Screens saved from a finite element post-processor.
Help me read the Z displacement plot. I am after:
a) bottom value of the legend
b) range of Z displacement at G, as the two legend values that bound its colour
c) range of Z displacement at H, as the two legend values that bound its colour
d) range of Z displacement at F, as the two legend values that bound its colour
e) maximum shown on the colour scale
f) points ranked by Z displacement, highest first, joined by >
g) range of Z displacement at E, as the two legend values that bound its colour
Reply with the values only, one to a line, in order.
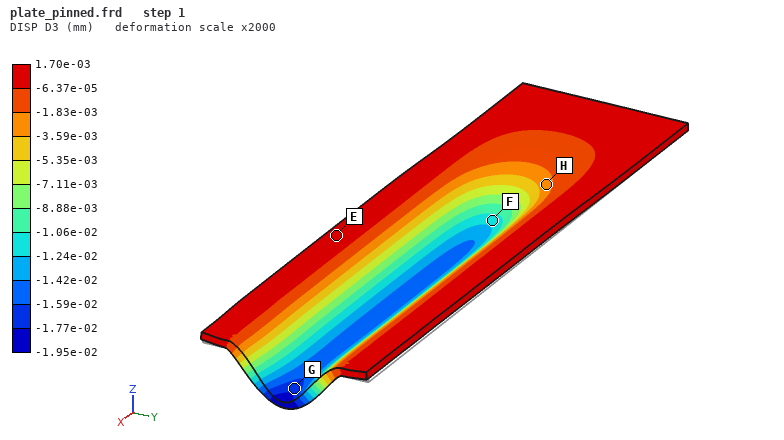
-1.95e-02 mm
-1.77e-02 to -1.59e-02 mm
-3.59e-03 to -1.83e-03 mm
-1.24e-02 to -1.06e-02 mm
1.70e-03 mm
E > H > F > G
-6.37e-05 to 1.70e-03 mm
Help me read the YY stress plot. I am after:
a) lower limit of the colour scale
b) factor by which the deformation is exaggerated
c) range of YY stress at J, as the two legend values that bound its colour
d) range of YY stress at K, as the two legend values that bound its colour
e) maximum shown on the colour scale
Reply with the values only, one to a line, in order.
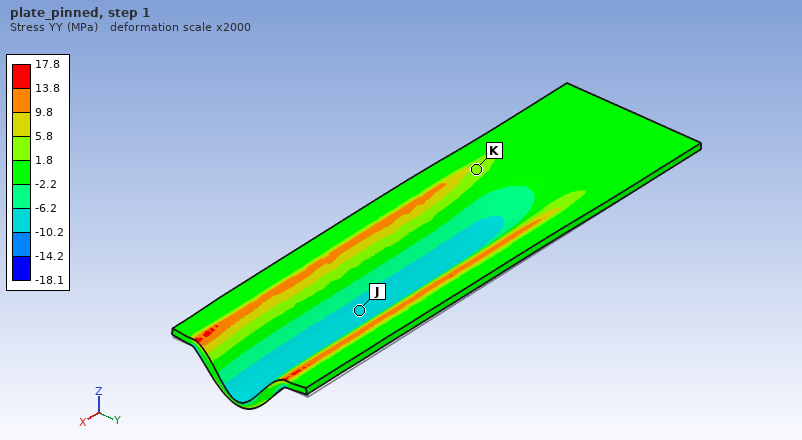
-18.1 MPa
2000
-10.2 to -6.2 MPa
1.8 to 5.8 MPa
17.8 MPa
